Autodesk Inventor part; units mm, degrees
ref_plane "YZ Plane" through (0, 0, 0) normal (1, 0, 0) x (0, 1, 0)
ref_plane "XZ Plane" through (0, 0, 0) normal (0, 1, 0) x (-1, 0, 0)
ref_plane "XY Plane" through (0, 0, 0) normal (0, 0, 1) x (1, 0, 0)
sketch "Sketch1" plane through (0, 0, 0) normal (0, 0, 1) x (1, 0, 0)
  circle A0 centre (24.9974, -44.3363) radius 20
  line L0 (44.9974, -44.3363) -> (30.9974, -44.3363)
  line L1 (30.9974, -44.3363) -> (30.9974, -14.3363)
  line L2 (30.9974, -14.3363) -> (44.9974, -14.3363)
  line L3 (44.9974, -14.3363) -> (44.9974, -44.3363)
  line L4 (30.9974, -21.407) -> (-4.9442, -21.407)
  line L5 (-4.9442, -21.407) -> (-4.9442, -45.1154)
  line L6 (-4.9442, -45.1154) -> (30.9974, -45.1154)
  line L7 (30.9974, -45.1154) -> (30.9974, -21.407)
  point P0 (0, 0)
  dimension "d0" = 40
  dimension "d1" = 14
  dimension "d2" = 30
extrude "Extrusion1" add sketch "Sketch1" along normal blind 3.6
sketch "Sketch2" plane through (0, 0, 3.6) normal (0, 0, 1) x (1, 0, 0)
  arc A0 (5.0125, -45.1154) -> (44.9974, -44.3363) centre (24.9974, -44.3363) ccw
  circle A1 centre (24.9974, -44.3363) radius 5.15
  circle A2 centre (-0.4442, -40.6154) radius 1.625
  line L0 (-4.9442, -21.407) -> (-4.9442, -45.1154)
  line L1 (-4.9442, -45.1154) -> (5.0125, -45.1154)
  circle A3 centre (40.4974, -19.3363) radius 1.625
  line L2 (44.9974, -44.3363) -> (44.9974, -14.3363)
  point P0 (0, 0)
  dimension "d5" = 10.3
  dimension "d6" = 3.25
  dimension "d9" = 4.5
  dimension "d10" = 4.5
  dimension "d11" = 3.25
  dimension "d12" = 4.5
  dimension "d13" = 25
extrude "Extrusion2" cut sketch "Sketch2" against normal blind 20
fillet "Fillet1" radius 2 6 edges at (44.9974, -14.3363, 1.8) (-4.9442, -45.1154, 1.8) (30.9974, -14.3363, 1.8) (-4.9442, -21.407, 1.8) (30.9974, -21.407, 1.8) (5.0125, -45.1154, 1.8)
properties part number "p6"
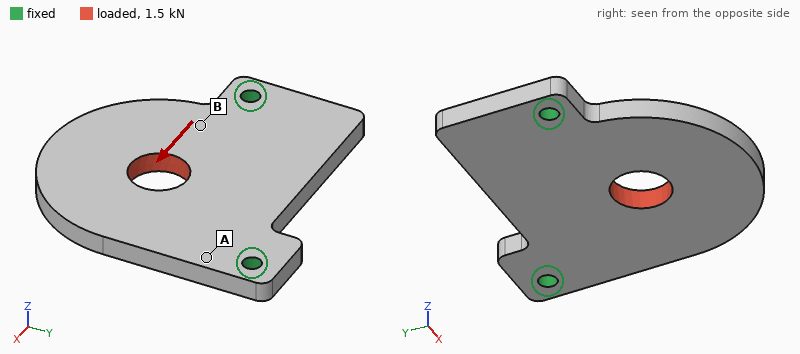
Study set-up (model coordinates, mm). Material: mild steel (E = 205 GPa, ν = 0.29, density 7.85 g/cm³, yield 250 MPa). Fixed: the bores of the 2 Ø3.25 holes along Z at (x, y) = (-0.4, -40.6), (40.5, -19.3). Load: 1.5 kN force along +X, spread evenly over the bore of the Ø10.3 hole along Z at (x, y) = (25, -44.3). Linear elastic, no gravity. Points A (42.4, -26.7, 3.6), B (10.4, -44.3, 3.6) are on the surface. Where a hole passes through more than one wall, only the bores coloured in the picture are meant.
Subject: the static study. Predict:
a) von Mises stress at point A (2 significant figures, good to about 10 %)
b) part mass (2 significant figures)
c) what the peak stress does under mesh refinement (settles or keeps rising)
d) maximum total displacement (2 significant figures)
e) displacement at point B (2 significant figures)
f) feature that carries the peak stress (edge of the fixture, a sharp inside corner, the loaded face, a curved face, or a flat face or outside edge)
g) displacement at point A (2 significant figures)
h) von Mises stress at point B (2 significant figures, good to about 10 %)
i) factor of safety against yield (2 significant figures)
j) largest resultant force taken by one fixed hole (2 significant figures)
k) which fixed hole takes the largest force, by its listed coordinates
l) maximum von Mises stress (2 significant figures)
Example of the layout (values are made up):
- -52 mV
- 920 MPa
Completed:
- 7.6 MPa
- 50 g
- settles
- 4.2 µm
- 1.7 µm
- a curved face
- 1.3 µm
- 27 MPa
- 2.6
- 1.2 kN
- (-0.4, -40.6)
- 95 MPa
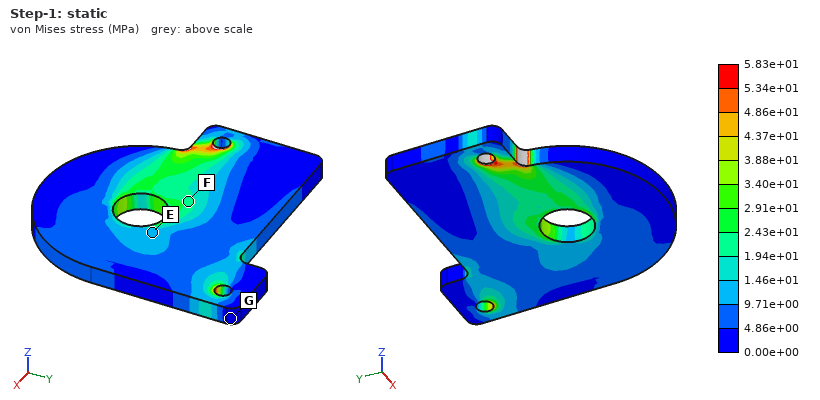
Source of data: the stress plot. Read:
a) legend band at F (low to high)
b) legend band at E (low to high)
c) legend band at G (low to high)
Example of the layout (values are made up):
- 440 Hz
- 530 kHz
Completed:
- 1.94e+01 to 2.43e+01 MPa
- 9.71e+00 to 1.46e+01 MPa
- 0.00e+00 to 4.86e+00 MPa
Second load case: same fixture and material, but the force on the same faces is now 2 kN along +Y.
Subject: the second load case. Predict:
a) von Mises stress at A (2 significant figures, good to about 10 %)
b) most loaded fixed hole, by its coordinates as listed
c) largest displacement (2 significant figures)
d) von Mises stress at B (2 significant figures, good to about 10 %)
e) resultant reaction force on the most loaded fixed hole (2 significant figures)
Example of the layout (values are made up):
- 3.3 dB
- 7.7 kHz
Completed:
- 32 MPa
- (40.5, -19.3)
- 4.3 µm
- 11 MPa
- 1.4 kN
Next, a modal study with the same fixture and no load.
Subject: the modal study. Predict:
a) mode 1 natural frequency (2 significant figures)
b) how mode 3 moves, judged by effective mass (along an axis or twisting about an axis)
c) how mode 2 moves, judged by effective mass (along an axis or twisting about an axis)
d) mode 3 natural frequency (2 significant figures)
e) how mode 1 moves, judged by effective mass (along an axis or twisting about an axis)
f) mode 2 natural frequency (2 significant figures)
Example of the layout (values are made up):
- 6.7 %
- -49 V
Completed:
- 2200 Hz
- along Z
- along Z
- 7600 Hz
- along Z
- 7000 Hz
